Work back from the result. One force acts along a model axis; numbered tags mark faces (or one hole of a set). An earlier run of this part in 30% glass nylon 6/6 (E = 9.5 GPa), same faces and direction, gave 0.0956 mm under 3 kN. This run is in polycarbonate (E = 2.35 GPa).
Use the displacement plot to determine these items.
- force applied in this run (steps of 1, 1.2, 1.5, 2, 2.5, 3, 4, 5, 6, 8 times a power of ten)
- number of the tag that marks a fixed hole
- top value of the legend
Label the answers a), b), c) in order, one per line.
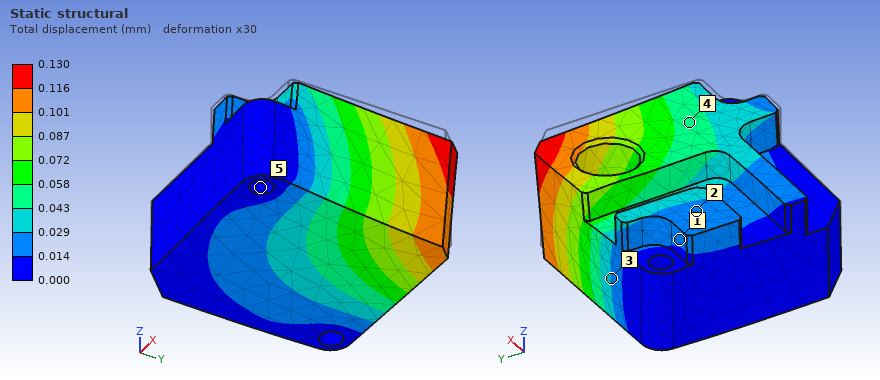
a) 1 kN
b) 5
c) 0.130 mm
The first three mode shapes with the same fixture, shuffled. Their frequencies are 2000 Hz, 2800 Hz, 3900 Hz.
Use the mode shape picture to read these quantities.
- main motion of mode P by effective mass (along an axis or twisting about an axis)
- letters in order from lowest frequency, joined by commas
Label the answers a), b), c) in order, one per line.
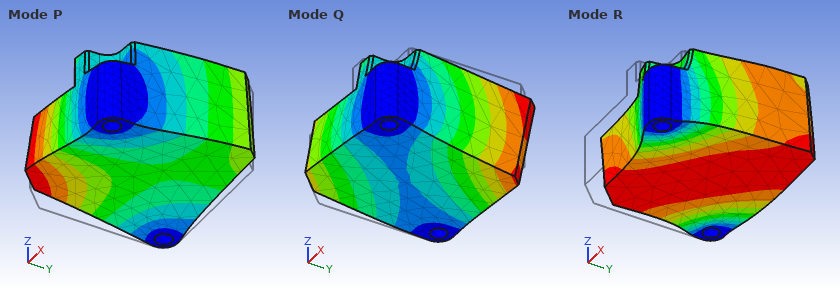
a) along Z
b) Q, P, R
